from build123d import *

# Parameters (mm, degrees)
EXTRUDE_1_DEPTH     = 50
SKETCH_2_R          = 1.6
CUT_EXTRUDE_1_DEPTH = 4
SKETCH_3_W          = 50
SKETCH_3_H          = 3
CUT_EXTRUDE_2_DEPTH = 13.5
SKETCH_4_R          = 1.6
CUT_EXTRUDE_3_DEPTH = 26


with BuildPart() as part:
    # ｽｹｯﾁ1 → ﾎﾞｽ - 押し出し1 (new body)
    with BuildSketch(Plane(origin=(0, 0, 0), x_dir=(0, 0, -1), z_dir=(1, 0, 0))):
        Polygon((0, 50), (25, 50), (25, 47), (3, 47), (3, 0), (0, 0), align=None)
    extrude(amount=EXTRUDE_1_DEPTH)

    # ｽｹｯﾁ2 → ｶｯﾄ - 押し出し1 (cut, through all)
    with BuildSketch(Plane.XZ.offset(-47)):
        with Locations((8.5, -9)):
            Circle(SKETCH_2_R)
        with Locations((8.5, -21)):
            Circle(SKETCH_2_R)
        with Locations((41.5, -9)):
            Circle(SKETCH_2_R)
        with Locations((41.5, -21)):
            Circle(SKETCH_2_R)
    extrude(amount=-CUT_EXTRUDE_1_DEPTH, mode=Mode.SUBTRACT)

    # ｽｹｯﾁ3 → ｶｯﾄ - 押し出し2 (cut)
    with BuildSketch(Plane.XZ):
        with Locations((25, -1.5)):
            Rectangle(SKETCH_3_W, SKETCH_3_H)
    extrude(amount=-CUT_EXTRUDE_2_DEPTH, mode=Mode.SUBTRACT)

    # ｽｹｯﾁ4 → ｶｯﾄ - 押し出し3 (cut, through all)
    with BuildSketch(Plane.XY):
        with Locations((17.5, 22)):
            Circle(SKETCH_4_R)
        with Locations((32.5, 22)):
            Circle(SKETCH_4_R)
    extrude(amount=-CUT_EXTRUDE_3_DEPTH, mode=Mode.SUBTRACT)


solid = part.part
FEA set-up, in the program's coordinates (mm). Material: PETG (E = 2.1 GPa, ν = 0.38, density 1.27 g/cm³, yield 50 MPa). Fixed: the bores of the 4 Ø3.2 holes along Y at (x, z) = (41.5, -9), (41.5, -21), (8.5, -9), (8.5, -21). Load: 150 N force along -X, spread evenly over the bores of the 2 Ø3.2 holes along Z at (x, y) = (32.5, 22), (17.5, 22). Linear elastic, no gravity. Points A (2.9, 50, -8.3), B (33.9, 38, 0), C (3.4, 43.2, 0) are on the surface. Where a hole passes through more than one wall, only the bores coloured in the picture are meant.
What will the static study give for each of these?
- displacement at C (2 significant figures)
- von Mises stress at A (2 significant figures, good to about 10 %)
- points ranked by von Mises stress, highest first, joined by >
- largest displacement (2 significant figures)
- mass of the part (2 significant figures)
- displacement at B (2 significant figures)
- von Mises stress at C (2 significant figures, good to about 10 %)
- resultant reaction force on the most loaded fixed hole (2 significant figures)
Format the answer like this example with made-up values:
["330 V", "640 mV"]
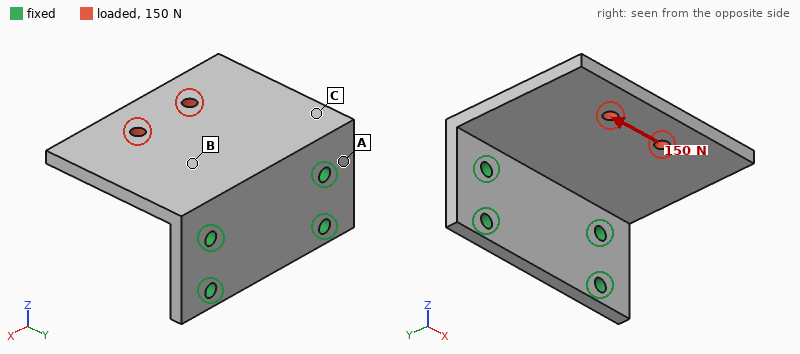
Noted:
["0.26 mm", "11 MPa", "A > C > B", "0.62 mm", "11 g", "0.16 mm", "4.0 MPa", "150 N"]
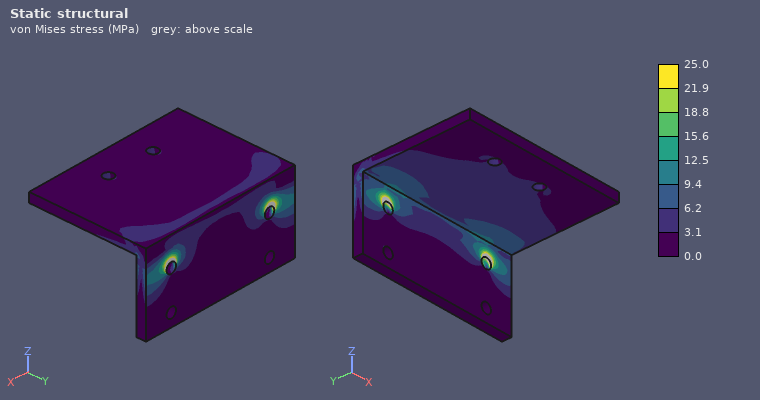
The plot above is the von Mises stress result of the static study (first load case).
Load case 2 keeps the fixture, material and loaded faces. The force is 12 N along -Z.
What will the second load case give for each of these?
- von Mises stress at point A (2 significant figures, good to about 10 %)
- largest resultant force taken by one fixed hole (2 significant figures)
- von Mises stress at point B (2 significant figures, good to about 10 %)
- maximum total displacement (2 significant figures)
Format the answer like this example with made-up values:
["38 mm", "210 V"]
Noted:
["2.6 MPa", "7.3 N", "2.3 MPa", "0.77 mm"]
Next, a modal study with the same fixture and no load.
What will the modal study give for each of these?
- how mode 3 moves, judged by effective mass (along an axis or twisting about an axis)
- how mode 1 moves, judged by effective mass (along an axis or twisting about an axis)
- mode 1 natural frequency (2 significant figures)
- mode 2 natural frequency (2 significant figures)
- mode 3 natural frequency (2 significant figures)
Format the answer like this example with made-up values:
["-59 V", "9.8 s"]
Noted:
["along X", "along Z", "400 Hz", "820 Hz", "1700 Hz"]
